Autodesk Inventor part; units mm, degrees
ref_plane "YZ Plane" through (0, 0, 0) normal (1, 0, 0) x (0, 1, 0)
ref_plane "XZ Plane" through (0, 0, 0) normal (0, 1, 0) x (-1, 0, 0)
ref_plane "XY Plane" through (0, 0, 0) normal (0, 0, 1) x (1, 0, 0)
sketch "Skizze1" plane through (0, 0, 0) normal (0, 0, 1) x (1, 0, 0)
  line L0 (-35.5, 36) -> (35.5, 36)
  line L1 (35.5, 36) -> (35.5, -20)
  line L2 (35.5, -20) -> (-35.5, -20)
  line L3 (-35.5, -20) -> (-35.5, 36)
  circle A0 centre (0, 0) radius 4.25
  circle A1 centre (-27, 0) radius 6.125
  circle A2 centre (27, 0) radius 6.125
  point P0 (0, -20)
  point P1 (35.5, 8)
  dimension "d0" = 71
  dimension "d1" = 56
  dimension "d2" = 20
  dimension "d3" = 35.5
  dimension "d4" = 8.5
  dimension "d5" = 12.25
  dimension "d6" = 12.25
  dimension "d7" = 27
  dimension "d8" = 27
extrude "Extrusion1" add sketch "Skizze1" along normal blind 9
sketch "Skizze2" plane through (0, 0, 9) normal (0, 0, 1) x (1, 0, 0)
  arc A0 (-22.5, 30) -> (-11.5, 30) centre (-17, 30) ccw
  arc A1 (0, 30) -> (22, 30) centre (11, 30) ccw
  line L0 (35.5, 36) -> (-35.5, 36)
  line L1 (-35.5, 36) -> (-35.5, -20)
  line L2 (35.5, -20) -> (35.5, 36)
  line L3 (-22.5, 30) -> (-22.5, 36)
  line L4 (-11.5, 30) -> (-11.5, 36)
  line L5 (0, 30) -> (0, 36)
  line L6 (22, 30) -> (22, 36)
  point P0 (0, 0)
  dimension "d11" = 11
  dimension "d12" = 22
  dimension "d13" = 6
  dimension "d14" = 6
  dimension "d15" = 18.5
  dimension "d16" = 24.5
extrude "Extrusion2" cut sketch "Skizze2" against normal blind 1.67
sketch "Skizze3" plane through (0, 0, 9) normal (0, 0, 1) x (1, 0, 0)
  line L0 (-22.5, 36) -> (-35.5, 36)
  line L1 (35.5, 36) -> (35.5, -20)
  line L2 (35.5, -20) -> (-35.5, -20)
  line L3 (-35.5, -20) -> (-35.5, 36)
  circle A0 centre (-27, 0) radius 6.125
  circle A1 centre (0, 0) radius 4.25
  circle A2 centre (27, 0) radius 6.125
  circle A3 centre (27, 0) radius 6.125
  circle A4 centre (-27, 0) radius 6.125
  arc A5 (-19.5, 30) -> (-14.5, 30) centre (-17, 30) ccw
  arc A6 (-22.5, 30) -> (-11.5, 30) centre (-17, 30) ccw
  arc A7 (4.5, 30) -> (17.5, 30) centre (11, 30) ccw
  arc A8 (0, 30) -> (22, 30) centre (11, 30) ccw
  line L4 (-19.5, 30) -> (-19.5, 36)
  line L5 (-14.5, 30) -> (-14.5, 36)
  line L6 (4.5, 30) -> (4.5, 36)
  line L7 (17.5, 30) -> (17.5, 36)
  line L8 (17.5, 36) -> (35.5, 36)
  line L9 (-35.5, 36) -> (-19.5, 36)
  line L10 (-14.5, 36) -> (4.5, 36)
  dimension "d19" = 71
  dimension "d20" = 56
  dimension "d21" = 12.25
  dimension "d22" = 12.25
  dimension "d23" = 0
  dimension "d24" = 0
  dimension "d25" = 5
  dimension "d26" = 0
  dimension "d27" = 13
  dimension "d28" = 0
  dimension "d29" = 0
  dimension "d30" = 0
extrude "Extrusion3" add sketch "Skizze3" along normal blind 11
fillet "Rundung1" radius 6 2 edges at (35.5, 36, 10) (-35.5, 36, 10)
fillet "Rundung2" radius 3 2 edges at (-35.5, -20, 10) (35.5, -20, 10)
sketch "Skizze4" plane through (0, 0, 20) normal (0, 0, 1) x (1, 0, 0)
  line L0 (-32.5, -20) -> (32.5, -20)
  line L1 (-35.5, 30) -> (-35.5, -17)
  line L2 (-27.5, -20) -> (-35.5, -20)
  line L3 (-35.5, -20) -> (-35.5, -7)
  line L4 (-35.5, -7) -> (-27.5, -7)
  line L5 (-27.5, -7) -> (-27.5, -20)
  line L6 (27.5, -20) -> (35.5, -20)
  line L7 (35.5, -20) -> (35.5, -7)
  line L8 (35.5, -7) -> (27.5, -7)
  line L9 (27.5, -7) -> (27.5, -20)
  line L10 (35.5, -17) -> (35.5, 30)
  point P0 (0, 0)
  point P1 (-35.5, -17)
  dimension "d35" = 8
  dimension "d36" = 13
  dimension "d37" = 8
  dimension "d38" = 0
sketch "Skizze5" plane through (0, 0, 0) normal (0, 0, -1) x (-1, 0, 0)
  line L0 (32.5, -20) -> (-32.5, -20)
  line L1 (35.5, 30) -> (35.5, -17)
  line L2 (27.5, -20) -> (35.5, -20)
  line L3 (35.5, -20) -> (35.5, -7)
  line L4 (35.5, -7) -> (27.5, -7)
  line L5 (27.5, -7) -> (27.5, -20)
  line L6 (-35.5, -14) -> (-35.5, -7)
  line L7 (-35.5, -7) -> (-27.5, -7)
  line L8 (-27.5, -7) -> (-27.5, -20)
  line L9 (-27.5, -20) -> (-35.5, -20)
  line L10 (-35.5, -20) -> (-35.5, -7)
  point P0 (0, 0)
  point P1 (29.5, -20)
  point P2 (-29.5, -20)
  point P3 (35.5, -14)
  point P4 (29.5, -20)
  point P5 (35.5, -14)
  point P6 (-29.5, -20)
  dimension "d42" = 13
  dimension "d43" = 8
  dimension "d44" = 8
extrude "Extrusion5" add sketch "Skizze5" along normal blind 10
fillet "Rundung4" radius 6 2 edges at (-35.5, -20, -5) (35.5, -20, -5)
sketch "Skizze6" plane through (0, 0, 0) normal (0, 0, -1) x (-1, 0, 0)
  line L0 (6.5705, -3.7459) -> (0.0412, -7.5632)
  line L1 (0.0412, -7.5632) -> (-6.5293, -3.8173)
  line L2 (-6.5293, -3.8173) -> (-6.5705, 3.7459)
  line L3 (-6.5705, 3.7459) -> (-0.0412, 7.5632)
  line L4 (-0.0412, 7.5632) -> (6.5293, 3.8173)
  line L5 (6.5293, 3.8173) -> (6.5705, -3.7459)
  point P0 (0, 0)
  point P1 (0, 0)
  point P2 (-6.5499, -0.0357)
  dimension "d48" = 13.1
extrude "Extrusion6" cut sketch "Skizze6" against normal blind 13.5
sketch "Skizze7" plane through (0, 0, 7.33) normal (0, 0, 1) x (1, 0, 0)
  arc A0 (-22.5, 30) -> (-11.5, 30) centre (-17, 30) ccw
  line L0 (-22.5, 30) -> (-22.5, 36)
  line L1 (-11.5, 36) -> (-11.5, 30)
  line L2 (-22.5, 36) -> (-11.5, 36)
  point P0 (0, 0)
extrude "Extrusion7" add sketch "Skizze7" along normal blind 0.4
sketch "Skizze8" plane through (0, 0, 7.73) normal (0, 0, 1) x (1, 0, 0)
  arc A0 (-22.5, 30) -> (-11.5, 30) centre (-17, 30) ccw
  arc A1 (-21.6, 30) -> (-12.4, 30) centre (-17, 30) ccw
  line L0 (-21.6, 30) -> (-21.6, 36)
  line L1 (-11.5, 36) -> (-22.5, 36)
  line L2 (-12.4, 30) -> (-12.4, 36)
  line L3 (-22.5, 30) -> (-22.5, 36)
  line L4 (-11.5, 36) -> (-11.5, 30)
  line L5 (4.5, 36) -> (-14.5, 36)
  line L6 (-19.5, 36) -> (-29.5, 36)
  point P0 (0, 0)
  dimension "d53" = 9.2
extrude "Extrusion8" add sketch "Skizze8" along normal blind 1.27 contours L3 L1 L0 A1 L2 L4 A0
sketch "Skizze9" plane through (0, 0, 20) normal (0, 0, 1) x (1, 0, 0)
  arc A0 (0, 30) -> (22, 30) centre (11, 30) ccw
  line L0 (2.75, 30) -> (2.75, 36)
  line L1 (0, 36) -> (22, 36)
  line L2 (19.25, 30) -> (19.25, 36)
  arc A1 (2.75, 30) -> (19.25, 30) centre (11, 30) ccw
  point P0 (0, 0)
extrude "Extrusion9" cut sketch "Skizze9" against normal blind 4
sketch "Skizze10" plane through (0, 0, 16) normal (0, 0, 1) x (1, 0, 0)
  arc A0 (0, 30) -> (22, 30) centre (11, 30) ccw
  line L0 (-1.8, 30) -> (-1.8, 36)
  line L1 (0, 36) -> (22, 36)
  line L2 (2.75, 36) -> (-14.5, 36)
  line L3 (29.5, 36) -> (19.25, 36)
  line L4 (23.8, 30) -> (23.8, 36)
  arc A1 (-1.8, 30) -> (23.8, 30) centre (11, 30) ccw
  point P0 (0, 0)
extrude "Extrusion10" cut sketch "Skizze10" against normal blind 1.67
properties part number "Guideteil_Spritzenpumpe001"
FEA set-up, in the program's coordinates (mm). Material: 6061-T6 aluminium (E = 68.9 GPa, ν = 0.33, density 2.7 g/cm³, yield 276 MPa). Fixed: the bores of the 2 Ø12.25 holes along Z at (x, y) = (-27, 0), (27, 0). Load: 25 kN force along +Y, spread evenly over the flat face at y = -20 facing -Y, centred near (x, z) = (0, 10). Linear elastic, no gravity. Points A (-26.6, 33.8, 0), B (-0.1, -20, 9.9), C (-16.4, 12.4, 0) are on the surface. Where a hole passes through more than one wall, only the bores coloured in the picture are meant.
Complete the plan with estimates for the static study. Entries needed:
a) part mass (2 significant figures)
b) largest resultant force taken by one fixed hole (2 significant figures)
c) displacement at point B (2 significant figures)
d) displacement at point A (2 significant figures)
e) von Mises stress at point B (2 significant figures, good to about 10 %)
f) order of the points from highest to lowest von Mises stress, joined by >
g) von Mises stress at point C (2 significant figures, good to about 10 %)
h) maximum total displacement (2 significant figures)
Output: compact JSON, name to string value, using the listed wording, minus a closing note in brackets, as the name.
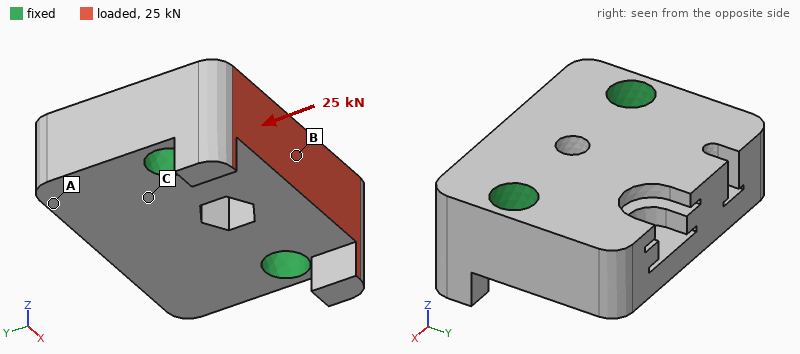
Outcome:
{"part mass": "190 g", "largest resultant force taken by one fixed hole": "13 kN", "displacement at point B": "13 µm", "displacement at point A": "2.3 µm", "von Mises stress at point B": "25 MPa", "order of the points from highest to lowest von Mises stress, joined by >": "B > C > A", "von Mises stress at point C": "12 MPa", "maximum total displacement": "14 µm"}
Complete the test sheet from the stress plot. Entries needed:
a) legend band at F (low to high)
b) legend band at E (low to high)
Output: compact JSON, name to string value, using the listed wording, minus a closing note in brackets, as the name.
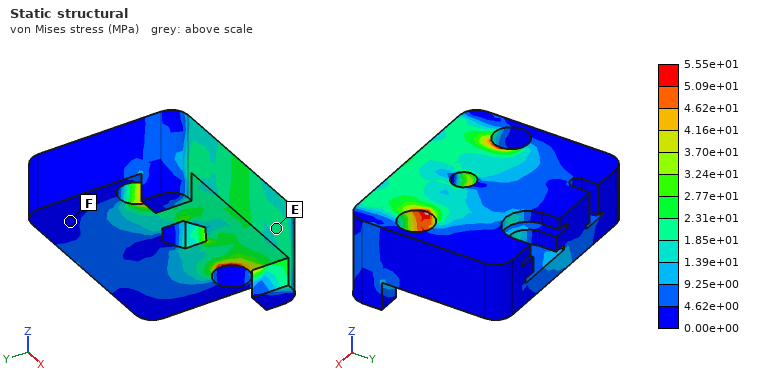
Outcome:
{"legend band at F": "0.00e+00 to 4.62e+00 MPa", "legend band at E": "1.85e+01 to 2.31e+01 MPa"}
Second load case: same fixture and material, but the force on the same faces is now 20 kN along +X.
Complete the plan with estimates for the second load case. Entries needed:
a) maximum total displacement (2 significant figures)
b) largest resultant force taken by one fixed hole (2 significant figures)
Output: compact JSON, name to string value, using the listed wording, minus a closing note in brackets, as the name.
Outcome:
{"maximum total displacement": "22 µm", "largest resultant force taken by one fixed hole": "11 kN"}
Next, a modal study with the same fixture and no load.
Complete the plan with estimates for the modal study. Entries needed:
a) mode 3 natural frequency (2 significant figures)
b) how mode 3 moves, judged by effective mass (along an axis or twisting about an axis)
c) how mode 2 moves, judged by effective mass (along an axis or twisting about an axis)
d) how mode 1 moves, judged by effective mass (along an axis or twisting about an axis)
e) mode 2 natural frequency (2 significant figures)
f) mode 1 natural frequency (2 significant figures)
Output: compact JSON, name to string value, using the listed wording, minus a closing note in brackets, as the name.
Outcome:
{"mode 3 natural frequency": "20 kHz", "how mode 3 moves, judged by effective mass": "along X", "how mode 2 moves, judged by effective mass": "twisting about Y", "how mode 1 moves, judged by effective mass": "along Z", "mode 2 natural frequency": "15 kHz", "mode 1 natural frequency": "11 kHz"}
